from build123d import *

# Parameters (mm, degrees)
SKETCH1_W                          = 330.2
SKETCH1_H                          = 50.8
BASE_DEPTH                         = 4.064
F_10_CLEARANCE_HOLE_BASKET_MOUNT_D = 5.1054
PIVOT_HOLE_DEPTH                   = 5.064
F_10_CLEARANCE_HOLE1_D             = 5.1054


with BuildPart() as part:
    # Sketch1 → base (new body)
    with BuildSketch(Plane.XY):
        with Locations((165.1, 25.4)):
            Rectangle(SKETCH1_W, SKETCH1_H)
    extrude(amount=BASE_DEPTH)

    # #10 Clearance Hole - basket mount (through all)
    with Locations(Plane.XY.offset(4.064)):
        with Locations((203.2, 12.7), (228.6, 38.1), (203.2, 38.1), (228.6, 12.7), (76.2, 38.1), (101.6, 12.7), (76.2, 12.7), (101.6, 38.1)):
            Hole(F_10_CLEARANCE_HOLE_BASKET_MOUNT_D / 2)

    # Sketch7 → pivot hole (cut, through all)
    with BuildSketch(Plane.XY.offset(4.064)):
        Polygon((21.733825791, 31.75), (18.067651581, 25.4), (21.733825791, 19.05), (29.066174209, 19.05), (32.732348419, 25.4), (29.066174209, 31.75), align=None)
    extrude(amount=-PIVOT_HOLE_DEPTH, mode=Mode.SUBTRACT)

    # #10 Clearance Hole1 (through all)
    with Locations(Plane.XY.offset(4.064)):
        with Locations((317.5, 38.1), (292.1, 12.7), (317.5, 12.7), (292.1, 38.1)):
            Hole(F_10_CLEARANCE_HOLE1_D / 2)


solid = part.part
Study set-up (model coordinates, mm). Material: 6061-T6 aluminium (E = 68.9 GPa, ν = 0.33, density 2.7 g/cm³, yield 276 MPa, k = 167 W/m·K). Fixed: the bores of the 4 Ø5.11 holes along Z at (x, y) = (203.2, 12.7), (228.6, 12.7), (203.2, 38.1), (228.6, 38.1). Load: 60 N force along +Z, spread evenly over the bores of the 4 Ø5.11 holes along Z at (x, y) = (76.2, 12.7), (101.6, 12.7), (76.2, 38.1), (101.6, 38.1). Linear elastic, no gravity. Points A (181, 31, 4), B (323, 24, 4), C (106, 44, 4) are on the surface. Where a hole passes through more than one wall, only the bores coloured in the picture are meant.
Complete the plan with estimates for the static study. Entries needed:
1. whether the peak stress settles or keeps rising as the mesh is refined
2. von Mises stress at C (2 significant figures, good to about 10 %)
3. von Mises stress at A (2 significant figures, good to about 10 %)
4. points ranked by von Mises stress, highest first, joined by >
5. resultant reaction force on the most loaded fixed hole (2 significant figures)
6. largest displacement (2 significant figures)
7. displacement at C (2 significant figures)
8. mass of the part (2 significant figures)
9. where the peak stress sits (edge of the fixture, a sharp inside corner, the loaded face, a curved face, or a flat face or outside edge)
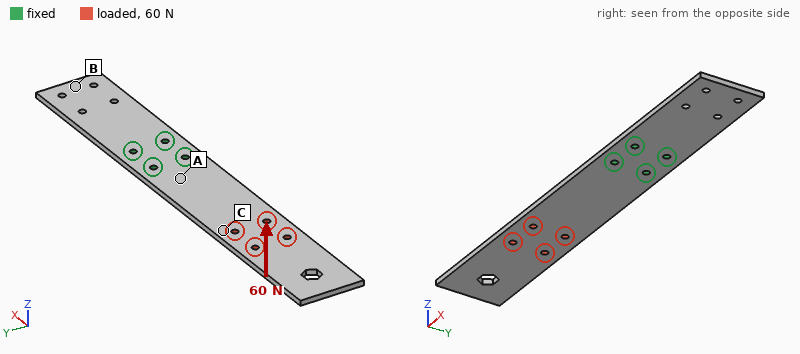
keeps rising
8.5 MPa
36 MPa
A > C > B
57 N
3.2 mm
1.1 mm
180 g
edge of the fixture
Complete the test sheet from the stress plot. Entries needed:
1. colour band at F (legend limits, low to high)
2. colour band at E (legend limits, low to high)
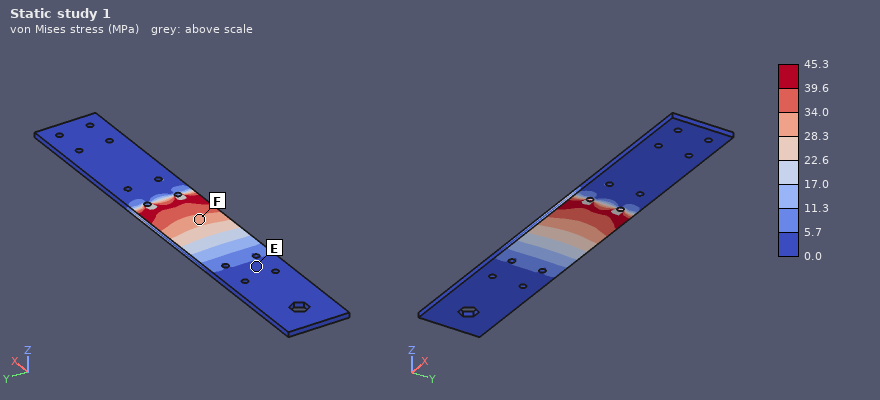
28.3 to 34.0 MPa
0.0 to 5.7 MPa
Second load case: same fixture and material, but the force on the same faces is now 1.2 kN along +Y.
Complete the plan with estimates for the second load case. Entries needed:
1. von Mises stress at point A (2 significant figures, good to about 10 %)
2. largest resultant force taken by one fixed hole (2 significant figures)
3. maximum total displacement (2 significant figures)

23 MPa
3.6 kN
0.52 mm
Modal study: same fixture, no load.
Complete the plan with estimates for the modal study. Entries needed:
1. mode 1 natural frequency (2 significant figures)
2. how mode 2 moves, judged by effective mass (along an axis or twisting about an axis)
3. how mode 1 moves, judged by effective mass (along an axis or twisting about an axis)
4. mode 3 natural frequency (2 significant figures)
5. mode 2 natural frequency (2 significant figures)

83 Hz
along Z
along Z
510 Hz
330 Hz
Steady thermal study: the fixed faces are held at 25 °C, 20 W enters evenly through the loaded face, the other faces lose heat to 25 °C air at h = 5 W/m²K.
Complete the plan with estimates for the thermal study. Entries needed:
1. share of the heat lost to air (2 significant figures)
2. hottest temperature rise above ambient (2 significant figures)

21 %
55 K
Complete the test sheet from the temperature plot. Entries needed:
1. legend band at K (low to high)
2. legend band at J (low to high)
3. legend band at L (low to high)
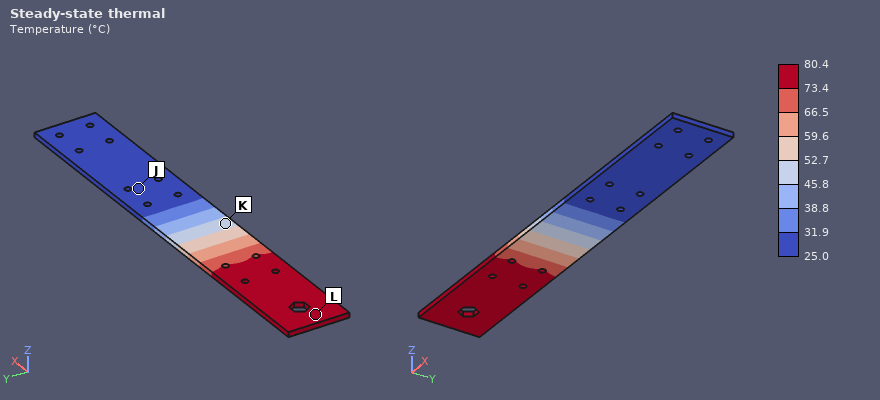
45.8 to 52.7 °C
25.0 to 31.9 °C
73.4 to 80.4 °C
